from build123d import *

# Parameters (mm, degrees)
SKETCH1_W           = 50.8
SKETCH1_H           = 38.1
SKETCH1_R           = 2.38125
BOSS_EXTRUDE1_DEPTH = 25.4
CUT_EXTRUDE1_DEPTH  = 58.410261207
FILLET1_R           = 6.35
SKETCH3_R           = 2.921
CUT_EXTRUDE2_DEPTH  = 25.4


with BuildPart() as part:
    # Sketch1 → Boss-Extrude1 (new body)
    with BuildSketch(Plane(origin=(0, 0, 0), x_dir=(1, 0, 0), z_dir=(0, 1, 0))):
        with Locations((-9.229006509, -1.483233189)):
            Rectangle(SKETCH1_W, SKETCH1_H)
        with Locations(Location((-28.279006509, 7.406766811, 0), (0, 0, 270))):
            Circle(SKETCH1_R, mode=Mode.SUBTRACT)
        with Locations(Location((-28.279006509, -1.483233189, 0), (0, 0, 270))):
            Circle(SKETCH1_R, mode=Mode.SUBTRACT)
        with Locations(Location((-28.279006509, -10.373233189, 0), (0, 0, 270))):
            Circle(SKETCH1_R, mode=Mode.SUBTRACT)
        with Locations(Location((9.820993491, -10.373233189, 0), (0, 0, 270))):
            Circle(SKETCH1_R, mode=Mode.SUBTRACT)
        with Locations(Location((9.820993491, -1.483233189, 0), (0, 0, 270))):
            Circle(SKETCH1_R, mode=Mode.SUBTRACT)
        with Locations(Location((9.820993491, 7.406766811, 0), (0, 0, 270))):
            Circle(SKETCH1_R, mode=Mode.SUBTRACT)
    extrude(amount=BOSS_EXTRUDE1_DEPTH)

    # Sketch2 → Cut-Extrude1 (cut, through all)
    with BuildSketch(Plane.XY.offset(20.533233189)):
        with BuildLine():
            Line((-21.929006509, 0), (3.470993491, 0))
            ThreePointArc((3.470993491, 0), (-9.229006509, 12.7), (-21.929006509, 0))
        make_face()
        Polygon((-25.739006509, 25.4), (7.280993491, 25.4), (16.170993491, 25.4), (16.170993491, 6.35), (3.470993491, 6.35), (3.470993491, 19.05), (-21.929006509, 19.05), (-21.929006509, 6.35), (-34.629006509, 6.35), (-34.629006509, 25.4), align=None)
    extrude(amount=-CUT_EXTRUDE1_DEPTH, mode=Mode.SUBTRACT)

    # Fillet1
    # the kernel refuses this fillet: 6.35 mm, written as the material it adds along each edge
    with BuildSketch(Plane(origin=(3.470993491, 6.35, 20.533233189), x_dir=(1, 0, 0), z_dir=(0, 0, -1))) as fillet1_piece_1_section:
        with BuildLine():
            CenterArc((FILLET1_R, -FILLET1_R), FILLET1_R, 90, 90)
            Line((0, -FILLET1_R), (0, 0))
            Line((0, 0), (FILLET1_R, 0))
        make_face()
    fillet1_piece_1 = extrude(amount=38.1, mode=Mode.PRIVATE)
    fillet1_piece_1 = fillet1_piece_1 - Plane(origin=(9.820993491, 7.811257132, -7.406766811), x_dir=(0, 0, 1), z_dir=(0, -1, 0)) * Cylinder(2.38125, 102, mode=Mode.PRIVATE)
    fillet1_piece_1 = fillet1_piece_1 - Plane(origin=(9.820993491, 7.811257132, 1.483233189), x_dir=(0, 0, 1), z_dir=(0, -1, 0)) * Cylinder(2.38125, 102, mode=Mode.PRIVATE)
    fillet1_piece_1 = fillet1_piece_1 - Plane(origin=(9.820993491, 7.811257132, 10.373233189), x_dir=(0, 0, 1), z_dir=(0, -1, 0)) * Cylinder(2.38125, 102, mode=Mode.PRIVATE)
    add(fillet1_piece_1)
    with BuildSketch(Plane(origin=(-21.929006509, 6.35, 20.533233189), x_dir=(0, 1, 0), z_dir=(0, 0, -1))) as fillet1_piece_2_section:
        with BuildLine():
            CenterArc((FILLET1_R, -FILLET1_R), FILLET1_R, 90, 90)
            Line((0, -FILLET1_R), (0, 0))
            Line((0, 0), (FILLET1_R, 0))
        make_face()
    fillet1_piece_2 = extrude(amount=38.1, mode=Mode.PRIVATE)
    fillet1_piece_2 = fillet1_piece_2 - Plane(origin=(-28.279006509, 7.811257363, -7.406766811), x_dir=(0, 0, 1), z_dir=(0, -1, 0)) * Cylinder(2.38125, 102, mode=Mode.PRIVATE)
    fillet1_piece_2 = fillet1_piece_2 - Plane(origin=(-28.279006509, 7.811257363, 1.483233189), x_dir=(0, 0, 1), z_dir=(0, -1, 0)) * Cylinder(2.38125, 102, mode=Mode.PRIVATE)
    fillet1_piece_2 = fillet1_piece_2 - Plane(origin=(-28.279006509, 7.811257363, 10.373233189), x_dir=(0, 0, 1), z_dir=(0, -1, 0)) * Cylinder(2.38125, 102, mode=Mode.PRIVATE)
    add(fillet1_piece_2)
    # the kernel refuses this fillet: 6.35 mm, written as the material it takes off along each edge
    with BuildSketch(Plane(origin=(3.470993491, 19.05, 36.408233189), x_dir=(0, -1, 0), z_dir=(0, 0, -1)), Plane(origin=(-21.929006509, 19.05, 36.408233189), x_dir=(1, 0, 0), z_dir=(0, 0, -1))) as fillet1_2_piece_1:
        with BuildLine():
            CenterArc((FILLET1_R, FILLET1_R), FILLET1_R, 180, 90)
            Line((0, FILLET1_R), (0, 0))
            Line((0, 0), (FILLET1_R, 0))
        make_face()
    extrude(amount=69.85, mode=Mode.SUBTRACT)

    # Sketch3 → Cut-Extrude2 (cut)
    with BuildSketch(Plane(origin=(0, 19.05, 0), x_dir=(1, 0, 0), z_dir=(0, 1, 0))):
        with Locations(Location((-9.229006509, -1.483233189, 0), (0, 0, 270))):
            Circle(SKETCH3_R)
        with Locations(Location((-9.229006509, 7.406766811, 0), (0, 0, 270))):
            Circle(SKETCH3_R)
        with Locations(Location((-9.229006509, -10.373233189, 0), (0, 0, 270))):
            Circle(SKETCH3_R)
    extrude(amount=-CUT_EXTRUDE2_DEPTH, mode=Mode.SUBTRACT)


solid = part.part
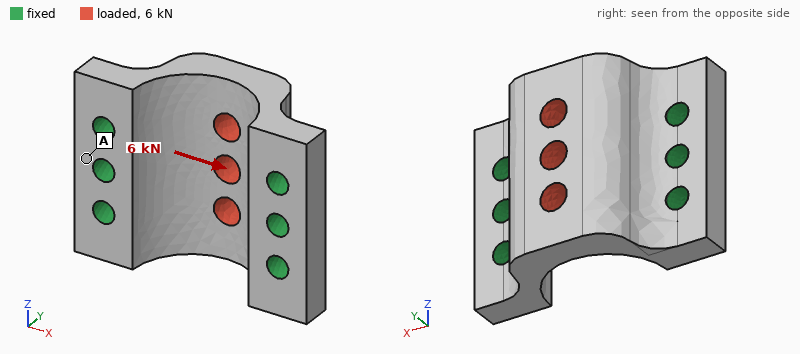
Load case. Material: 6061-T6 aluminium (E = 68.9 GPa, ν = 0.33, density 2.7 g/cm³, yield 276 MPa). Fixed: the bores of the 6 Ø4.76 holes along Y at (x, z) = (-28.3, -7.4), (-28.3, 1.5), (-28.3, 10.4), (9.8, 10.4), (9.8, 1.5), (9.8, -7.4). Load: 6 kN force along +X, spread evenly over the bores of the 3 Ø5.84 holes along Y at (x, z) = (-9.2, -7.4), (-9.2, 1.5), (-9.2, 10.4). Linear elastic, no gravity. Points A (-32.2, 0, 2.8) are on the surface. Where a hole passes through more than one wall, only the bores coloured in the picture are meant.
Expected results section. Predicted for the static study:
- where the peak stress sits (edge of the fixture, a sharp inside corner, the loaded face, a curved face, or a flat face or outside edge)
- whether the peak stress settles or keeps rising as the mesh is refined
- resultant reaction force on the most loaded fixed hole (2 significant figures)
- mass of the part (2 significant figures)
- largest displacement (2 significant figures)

edge of the fixture
keeps rising
1.3 kN
37 g
15 µm
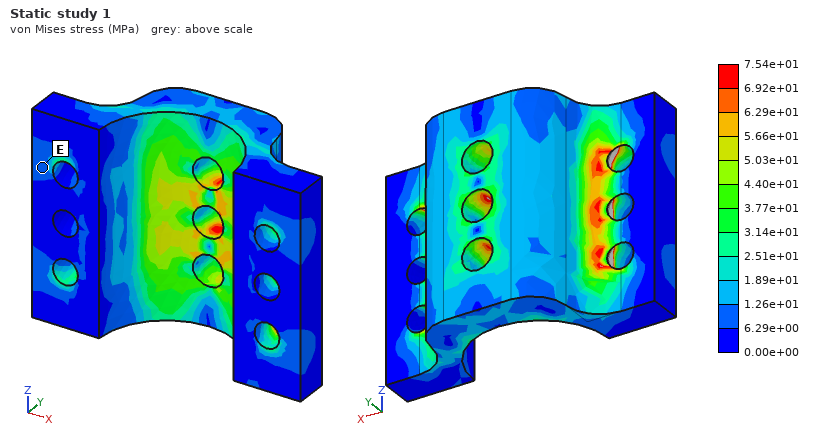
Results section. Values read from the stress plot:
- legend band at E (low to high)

6.29e+00 to 1.26e+01 MPa
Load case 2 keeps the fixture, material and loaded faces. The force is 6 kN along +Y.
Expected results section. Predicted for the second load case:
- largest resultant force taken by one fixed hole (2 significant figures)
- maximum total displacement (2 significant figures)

1.5 kN
21 µm
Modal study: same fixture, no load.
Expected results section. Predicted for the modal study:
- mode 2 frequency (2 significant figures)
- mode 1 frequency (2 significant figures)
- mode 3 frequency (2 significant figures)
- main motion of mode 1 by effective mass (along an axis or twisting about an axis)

25 kHz
18 kHz
26 kHz
along Z
